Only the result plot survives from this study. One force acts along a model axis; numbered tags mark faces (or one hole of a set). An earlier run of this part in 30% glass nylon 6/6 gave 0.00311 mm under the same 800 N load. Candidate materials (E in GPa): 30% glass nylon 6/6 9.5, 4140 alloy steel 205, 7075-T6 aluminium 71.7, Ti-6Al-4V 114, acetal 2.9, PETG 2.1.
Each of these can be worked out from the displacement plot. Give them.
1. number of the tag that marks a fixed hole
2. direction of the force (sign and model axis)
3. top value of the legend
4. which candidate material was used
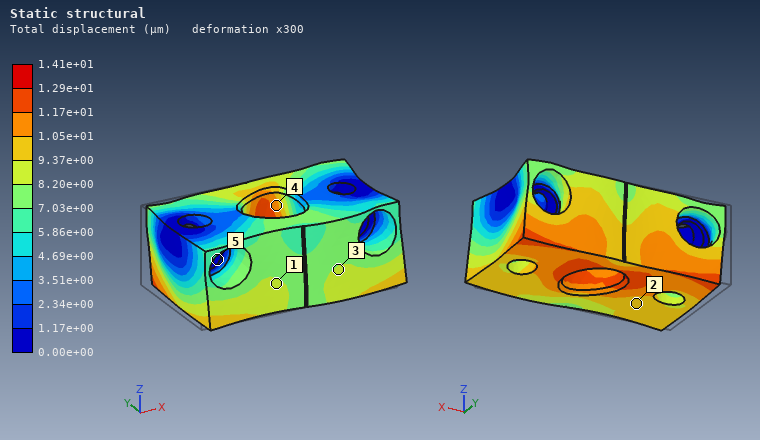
5
+X
1.41e+01 µm
PETG
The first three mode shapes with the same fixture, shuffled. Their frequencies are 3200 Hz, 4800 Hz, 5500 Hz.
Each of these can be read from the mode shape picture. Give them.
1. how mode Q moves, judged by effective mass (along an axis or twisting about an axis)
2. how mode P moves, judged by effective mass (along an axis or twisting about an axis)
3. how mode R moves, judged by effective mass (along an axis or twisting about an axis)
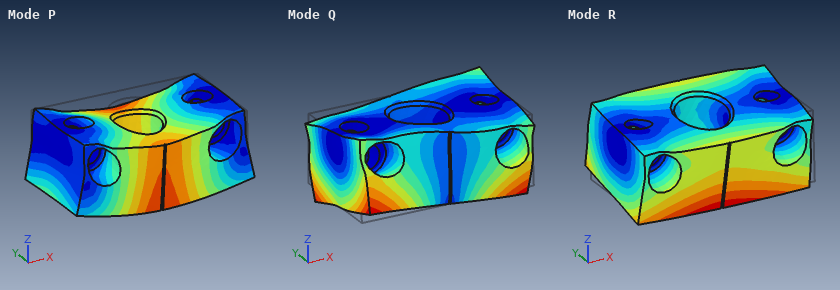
twisting about Z
along Z
along Y
